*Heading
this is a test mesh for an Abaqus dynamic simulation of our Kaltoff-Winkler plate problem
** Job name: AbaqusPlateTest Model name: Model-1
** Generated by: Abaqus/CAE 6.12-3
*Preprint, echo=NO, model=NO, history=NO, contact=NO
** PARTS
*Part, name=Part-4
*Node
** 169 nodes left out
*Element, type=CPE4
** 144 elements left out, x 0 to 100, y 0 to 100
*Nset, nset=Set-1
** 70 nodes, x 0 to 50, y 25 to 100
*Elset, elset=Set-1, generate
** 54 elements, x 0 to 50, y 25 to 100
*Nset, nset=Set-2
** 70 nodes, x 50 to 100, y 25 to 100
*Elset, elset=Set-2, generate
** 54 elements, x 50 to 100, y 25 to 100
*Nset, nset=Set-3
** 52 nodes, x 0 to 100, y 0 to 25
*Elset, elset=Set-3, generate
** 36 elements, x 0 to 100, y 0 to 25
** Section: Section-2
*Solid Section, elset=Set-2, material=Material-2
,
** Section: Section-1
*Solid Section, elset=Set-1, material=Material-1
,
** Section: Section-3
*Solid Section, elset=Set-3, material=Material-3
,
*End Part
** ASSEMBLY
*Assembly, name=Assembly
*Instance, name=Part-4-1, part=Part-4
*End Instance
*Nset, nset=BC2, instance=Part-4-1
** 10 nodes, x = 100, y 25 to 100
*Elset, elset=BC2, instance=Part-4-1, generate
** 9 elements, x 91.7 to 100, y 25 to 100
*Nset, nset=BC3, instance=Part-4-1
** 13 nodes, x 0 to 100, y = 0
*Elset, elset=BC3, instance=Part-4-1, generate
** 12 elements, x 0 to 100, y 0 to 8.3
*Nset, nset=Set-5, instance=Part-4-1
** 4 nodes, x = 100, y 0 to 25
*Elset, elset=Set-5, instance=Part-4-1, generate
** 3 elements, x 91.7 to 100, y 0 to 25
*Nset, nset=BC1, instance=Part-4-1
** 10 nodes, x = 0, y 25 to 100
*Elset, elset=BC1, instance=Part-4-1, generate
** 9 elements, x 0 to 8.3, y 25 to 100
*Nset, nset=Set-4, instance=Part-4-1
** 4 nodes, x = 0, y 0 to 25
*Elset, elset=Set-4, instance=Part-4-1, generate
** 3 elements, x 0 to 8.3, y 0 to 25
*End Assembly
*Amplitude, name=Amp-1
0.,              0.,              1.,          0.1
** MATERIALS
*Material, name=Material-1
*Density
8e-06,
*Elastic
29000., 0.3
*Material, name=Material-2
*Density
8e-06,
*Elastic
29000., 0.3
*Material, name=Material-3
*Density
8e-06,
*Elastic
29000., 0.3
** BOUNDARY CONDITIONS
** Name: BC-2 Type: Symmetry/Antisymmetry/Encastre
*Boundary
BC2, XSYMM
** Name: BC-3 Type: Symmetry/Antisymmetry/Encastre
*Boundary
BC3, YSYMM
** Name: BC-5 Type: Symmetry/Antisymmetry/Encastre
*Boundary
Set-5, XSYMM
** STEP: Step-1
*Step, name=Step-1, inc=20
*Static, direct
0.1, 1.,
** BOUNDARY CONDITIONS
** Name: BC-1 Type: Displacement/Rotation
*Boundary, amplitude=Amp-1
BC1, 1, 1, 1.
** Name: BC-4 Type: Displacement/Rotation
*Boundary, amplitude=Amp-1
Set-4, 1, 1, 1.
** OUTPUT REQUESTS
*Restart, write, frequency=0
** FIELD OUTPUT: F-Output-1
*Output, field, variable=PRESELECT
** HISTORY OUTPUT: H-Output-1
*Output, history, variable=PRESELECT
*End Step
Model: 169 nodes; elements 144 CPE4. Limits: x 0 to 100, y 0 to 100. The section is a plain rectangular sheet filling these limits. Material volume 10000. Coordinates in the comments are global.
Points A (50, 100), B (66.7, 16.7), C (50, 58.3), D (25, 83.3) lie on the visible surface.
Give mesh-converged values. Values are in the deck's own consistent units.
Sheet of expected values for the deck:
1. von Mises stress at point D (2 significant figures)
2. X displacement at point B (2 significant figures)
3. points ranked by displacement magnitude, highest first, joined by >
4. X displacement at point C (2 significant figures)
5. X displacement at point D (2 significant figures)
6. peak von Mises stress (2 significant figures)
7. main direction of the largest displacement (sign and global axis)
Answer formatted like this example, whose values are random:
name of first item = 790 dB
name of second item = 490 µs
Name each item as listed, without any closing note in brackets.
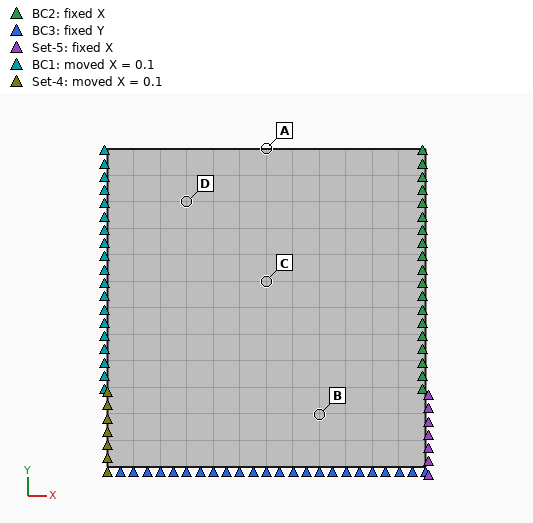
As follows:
von Mises stress at point D = 28
X displacement at point B = 0.033
points ranked by displacement magnitude, highest first, joined by > = D > A > C > B
X displacement at point C = 0.050
X displacement at point D = 0.075
peak von Mises stress = 28
main direction of the largest displacement = +X
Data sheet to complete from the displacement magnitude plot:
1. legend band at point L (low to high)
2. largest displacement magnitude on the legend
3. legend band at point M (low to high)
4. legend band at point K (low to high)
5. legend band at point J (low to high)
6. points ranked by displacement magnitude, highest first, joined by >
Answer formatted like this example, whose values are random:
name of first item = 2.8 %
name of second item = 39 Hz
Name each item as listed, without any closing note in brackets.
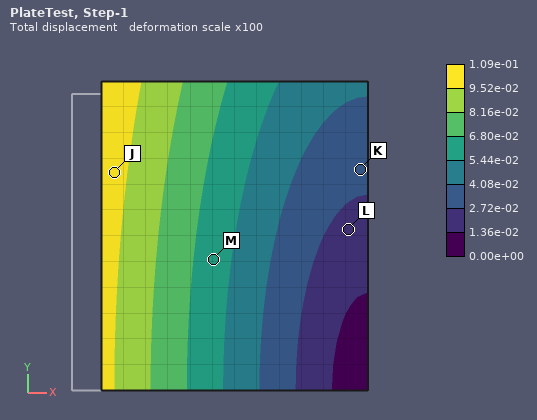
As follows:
legend band at point L = 1.36e-02 to 2.72e-02
largest displacement magnitude on the legend = 1.09e-01
legend band at point M = 5.44e-02 to 6.80e-02
legend band at point K = 2.72e-02 to 4.08e-02
legend band at point J = 9.52e-02 to 1.09e-01
points ranked by displacement magnitude, highest first, joined by > = J > M > K > L
